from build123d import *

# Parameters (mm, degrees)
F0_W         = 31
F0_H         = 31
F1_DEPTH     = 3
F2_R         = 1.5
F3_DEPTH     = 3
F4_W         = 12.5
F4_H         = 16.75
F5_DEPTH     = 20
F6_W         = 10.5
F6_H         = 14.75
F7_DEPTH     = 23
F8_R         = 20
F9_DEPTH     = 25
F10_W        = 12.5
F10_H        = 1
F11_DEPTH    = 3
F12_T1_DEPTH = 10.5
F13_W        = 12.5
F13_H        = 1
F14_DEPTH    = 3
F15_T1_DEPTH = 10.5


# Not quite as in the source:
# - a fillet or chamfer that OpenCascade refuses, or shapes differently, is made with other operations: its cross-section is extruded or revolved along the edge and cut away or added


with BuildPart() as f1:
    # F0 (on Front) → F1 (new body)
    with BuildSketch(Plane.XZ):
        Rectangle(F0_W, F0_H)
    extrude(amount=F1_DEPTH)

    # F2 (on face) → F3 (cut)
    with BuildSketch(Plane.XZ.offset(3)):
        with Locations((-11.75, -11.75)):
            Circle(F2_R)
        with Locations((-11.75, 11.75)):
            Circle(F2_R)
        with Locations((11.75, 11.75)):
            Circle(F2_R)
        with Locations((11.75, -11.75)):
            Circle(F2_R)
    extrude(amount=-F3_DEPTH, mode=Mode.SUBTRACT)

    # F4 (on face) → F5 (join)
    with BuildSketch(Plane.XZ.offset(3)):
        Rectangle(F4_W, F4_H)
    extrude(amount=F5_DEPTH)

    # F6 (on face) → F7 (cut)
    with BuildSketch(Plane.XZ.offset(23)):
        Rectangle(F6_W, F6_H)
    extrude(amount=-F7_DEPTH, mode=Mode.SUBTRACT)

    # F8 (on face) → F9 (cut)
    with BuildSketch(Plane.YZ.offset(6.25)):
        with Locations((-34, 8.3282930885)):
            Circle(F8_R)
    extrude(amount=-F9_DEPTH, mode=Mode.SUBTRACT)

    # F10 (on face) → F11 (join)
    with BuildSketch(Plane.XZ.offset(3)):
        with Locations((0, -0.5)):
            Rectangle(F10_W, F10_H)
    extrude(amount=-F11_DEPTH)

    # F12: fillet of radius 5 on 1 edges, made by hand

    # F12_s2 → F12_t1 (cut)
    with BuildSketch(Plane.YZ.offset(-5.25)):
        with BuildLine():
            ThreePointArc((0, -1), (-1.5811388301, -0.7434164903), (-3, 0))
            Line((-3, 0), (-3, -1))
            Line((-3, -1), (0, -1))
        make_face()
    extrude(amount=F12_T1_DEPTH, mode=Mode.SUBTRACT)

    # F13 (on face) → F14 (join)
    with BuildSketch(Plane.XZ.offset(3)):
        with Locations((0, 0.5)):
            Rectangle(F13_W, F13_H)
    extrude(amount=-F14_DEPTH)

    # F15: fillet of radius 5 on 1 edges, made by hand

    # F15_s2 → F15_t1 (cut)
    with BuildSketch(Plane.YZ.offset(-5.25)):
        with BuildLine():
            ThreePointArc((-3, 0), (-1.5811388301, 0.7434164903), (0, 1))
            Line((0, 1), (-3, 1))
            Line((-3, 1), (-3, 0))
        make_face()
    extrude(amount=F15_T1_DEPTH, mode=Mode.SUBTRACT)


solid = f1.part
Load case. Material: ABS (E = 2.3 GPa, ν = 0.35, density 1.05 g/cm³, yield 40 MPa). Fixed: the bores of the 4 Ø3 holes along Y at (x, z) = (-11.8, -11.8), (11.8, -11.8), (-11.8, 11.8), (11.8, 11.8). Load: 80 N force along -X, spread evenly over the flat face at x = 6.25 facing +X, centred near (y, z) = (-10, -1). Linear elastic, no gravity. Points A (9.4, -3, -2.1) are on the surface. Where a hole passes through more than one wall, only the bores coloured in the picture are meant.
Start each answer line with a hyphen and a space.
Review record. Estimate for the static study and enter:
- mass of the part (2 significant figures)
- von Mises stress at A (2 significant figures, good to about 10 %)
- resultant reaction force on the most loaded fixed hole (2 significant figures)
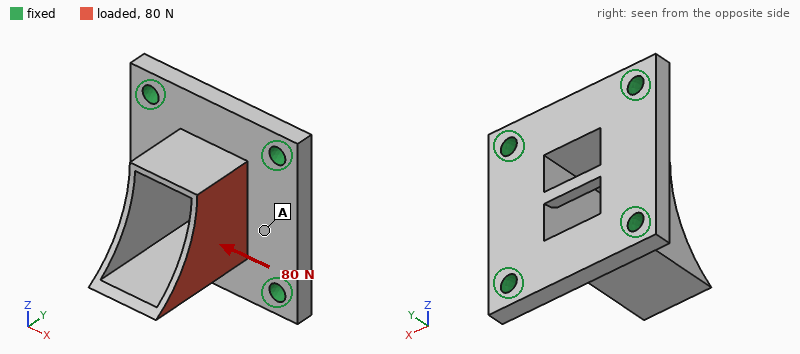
- 3.3 g
- 3.2 MPa
- 35 N
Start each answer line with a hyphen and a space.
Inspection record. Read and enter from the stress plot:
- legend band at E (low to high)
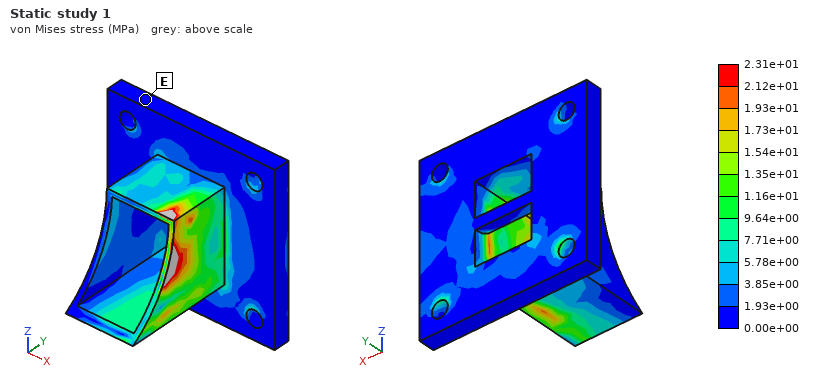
- 0.00e+00 to 1.93e+00 MPa
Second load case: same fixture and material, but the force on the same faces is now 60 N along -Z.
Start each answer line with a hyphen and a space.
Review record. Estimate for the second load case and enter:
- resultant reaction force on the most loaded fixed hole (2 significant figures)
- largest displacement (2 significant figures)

- 34 N
- 0.15 mm
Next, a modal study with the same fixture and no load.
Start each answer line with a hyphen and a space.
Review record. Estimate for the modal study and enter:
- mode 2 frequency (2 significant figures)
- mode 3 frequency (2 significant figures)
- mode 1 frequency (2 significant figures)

- 4400 Hz
- 5300 Hz
- 4100 Hz
